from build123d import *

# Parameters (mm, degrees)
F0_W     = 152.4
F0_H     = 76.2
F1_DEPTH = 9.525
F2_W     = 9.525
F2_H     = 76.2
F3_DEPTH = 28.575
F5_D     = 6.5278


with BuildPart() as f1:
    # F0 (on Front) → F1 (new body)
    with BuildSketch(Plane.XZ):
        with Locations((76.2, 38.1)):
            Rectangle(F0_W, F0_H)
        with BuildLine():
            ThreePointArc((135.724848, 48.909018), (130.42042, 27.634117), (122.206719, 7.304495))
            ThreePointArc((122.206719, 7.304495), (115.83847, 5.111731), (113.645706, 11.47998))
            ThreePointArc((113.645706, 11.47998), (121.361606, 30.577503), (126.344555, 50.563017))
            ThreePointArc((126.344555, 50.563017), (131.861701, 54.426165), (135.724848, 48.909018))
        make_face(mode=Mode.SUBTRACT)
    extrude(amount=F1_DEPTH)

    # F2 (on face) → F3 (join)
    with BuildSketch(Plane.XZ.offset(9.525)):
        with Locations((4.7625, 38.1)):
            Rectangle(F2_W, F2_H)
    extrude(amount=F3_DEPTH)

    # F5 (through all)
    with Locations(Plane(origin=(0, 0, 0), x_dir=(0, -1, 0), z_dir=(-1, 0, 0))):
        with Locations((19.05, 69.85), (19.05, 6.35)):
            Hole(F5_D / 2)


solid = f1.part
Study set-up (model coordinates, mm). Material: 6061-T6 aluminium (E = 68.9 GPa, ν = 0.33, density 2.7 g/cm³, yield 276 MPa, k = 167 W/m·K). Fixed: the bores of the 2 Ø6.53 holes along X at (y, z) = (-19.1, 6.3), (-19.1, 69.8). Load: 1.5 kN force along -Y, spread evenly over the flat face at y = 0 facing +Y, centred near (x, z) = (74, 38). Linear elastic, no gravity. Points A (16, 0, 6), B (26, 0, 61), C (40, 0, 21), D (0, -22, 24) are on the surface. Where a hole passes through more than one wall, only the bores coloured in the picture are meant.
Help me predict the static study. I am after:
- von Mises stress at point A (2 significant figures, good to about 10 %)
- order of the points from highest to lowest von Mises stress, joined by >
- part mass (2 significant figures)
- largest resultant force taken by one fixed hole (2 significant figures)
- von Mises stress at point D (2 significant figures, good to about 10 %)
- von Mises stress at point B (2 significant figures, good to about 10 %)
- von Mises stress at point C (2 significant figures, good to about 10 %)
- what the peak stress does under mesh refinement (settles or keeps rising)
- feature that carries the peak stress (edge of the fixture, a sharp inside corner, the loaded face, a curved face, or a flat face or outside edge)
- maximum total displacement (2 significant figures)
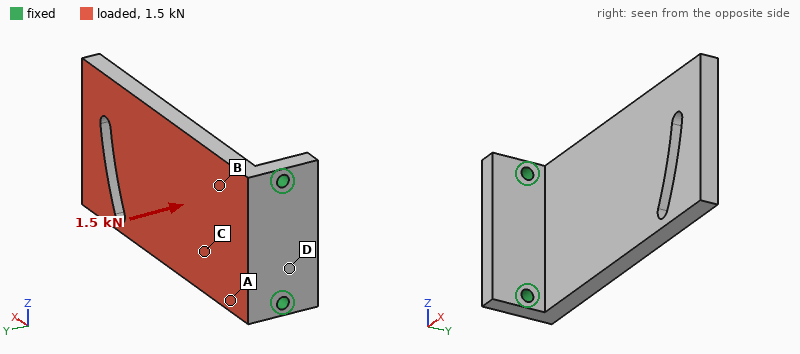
81 MPa
A > B > C > D
340 g
790 N
29 MPa
62 MPa
47 MPa
keeps rising
edge of the fixture
2.1 mm
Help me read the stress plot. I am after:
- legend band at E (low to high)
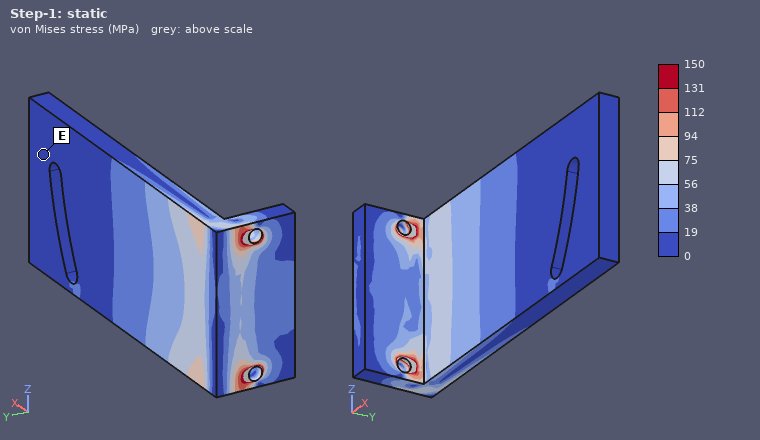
0 to 19 MPa
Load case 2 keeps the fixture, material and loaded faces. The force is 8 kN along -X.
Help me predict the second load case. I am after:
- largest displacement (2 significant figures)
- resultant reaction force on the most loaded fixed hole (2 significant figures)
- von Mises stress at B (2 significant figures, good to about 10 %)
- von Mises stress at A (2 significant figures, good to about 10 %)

1.4 mm
4.1 kN
37 MPa
46 MPa
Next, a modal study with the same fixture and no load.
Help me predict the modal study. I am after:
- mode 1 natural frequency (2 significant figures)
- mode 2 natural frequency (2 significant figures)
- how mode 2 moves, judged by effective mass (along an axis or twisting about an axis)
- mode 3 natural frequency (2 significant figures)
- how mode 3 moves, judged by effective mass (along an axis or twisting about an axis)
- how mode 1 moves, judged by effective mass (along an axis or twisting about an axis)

320 Hz
1300 Hz
along Z
1600 Hz
along Z
along Y
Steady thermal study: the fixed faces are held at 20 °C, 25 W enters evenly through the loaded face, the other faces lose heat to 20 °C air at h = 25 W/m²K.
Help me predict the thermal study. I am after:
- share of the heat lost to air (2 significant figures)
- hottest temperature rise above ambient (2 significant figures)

18 %
15 K
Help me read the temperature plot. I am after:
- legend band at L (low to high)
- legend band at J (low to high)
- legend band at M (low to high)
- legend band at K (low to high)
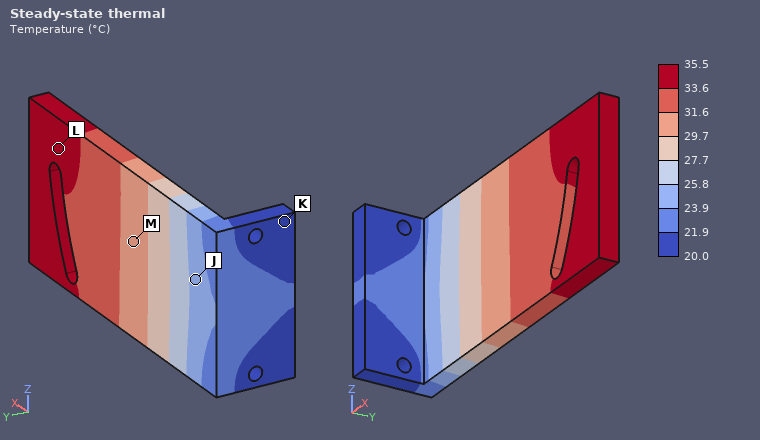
33.6 to 35.5 °C
23.9 to 25.8 °C
29.7 to 31.6 °C
20.0 to 21.9 °C
